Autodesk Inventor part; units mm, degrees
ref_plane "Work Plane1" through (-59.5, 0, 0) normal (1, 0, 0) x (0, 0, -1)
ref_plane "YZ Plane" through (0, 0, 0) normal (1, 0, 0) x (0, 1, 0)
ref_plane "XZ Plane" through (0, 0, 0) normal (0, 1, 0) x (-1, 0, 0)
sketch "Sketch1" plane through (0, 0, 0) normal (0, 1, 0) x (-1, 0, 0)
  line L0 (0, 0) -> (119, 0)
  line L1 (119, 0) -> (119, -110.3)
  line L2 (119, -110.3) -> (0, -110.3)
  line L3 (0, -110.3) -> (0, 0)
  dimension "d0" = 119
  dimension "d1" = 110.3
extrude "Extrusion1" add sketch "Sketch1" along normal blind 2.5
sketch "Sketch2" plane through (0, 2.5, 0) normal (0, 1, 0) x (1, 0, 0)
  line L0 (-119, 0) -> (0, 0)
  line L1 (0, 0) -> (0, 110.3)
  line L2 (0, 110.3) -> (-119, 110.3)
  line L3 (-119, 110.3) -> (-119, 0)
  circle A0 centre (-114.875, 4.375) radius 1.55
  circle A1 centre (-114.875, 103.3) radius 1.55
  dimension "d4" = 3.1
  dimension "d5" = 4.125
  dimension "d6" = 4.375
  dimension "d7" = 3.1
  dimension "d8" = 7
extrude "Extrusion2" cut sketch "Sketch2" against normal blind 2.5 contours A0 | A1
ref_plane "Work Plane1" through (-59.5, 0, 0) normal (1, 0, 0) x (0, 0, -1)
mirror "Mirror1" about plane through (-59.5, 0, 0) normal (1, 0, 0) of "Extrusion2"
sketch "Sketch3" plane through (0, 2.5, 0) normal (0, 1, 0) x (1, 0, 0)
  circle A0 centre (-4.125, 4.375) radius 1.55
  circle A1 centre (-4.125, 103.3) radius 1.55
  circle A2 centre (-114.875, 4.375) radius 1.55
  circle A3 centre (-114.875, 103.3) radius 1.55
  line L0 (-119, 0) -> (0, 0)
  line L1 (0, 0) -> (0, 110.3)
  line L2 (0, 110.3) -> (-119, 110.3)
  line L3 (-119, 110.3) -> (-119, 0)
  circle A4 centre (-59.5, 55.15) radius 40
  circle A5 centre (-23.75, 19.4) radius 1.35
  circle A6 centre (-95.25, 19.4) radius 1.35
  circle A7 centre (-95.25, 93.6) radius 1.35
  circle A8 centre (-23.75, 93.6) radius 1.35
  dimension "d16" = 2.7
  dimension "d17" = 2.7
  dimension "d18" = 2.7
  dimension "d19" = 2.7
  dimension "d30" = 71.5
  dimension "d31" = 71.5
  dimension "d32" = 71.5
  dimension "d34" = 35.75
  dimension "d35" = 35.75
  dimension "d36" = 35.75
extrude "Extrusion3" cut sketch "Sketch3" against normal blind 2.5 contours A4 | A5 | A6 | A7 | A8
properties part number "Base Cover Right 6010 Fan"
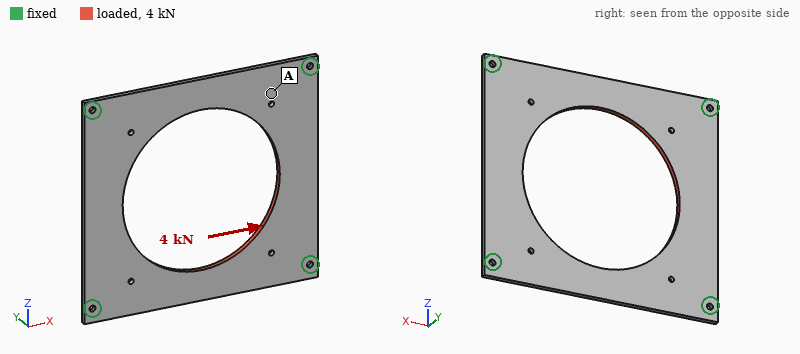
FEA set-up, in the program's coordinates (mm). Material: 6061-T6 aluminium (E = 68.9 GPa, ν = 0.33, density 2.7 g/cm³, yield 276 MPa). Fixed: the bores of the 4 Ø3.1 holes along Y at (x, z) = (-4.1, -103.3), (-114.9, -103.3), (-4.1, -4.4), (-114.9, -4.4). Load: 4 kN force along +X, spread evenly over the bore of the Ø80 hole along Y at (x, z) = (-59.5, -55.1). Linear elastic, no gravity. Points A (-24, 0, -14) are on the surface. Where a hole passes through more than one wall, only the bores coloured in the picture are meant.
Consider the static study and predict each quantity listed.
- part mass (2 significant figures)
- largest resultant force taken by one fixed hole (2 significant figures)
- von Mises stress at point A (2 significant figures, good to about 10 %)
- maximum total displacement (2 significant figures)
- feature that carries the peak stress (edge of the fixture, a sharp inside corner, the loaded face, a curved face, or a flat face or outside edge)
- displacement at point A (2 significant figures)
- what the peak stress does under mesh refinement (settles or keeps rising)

54 g
1.1 kN
9.5 MPa
39 µm
edge of the fixture
16 µm
keeps rising
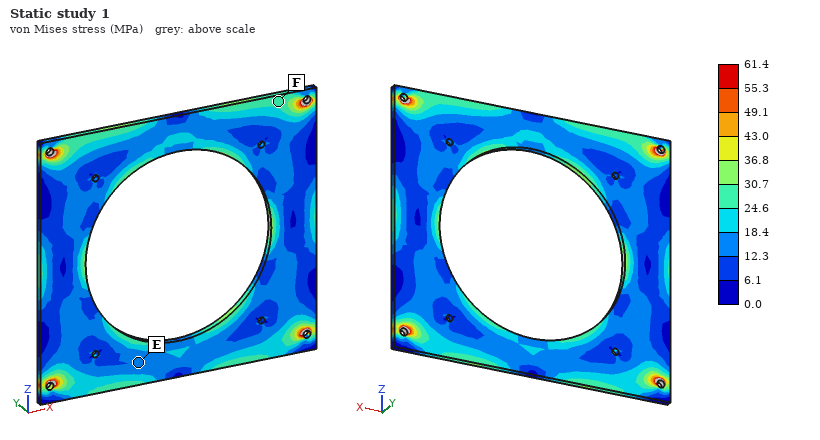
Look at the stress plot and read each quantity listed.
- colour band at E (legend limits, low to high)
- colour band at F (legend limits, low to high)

12.3 to 18.4 MPa
24.6 to 30.7 MPa
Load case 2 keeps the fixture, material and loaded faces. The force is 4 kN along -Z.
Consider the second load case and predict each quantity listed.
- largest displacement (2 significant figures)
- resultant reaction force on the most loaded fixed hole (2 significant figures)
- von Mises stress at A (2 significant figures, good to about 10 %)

51 µm
1.1 kN
11 MPa
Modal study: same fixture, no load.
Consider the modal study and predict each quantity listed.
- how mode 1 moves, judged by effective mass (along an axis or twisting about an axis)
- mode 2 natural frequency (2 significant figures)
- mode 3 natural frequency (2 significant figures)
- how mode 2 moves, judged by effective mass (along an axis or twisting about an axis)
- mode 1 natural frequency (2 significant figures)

along Y
1200 Hz
1300 Hz
twisting about X
970 Hz
